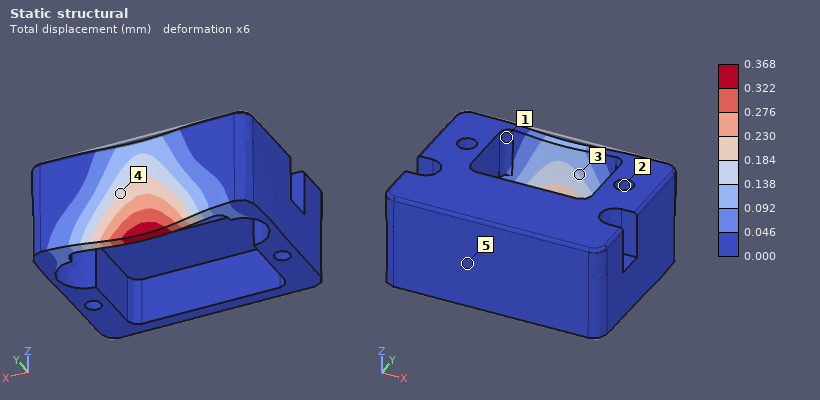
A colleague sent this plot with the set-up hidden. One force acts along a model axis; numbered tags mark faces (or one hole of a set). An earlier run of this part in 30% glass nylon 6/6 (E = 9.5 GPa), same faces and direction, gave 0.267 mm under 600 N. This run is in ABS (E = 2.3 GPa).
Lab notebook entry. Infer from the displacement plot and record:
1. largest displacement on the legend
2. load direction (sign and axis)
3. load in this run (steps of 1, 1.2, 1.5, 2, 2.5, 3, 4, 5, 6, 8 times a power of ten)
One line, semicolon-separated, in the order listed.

0.368 mm; -Y; 200 N
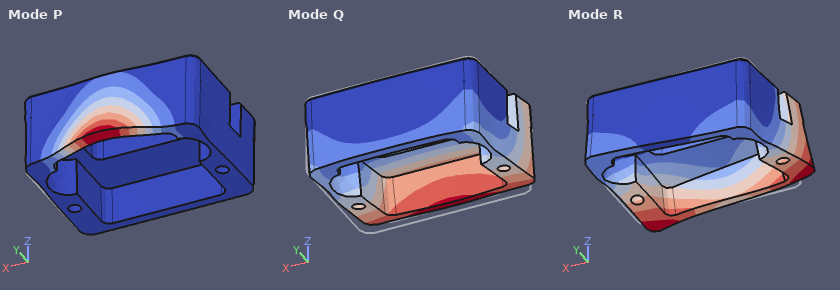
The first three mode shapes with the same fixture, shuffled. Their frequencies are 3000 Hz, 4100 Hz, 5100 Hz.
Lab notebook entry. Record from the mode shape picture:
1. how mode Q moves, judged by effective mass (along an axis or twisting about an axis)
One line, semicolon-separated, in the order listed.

along Z
